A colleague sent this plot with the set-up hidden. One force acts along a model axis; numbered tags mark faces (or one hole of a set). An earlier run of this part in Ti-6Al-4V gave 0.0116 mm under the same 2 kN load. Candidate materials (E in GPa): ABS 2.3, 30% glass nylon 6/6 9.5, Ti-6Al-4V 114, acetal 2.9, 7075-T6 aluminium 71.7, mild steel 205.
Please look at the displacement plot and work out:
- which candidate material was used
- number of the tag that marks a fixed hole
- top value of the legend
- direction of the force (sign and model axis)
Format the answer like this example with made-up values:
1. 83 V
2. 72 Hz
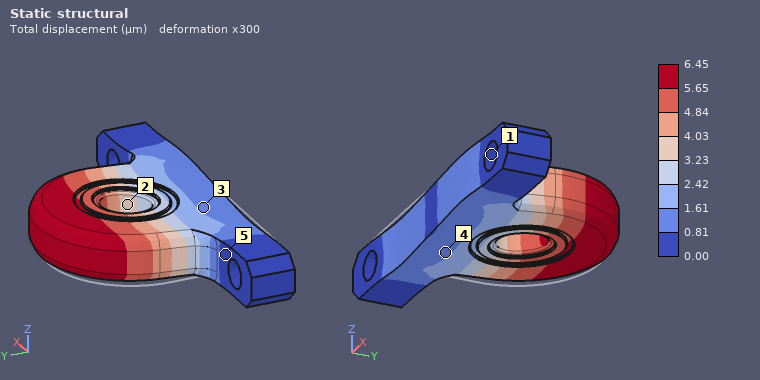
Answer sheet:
1. mild steel
2. 1
3. 6.45 µm
4. +X
